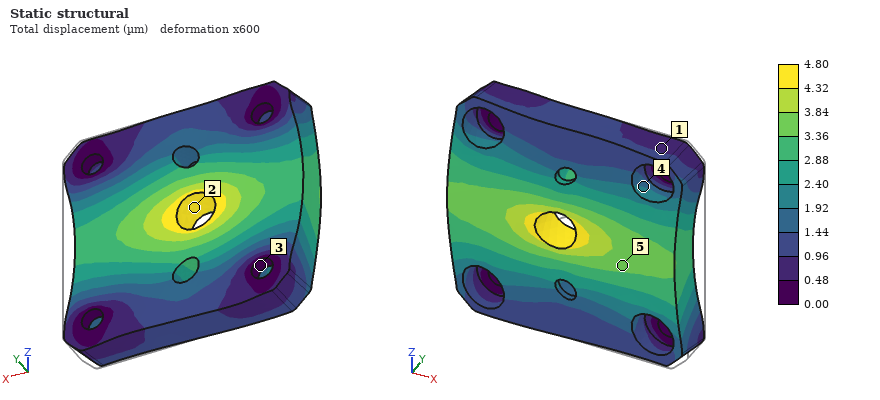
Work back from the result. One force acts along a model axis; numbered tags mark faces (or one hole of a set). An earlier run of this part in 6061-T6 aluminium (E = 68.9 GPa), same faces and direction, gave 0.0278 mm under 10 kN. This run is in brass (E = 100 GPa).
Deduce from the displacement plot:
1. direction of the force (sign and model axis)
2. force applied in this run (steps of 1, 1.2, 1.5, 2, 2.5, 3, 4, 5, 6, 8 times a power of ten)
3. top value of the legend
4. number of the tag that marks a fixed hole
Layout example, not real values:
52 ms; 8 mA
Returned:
-X; 2.5 kN; 4.80 µm; 3
